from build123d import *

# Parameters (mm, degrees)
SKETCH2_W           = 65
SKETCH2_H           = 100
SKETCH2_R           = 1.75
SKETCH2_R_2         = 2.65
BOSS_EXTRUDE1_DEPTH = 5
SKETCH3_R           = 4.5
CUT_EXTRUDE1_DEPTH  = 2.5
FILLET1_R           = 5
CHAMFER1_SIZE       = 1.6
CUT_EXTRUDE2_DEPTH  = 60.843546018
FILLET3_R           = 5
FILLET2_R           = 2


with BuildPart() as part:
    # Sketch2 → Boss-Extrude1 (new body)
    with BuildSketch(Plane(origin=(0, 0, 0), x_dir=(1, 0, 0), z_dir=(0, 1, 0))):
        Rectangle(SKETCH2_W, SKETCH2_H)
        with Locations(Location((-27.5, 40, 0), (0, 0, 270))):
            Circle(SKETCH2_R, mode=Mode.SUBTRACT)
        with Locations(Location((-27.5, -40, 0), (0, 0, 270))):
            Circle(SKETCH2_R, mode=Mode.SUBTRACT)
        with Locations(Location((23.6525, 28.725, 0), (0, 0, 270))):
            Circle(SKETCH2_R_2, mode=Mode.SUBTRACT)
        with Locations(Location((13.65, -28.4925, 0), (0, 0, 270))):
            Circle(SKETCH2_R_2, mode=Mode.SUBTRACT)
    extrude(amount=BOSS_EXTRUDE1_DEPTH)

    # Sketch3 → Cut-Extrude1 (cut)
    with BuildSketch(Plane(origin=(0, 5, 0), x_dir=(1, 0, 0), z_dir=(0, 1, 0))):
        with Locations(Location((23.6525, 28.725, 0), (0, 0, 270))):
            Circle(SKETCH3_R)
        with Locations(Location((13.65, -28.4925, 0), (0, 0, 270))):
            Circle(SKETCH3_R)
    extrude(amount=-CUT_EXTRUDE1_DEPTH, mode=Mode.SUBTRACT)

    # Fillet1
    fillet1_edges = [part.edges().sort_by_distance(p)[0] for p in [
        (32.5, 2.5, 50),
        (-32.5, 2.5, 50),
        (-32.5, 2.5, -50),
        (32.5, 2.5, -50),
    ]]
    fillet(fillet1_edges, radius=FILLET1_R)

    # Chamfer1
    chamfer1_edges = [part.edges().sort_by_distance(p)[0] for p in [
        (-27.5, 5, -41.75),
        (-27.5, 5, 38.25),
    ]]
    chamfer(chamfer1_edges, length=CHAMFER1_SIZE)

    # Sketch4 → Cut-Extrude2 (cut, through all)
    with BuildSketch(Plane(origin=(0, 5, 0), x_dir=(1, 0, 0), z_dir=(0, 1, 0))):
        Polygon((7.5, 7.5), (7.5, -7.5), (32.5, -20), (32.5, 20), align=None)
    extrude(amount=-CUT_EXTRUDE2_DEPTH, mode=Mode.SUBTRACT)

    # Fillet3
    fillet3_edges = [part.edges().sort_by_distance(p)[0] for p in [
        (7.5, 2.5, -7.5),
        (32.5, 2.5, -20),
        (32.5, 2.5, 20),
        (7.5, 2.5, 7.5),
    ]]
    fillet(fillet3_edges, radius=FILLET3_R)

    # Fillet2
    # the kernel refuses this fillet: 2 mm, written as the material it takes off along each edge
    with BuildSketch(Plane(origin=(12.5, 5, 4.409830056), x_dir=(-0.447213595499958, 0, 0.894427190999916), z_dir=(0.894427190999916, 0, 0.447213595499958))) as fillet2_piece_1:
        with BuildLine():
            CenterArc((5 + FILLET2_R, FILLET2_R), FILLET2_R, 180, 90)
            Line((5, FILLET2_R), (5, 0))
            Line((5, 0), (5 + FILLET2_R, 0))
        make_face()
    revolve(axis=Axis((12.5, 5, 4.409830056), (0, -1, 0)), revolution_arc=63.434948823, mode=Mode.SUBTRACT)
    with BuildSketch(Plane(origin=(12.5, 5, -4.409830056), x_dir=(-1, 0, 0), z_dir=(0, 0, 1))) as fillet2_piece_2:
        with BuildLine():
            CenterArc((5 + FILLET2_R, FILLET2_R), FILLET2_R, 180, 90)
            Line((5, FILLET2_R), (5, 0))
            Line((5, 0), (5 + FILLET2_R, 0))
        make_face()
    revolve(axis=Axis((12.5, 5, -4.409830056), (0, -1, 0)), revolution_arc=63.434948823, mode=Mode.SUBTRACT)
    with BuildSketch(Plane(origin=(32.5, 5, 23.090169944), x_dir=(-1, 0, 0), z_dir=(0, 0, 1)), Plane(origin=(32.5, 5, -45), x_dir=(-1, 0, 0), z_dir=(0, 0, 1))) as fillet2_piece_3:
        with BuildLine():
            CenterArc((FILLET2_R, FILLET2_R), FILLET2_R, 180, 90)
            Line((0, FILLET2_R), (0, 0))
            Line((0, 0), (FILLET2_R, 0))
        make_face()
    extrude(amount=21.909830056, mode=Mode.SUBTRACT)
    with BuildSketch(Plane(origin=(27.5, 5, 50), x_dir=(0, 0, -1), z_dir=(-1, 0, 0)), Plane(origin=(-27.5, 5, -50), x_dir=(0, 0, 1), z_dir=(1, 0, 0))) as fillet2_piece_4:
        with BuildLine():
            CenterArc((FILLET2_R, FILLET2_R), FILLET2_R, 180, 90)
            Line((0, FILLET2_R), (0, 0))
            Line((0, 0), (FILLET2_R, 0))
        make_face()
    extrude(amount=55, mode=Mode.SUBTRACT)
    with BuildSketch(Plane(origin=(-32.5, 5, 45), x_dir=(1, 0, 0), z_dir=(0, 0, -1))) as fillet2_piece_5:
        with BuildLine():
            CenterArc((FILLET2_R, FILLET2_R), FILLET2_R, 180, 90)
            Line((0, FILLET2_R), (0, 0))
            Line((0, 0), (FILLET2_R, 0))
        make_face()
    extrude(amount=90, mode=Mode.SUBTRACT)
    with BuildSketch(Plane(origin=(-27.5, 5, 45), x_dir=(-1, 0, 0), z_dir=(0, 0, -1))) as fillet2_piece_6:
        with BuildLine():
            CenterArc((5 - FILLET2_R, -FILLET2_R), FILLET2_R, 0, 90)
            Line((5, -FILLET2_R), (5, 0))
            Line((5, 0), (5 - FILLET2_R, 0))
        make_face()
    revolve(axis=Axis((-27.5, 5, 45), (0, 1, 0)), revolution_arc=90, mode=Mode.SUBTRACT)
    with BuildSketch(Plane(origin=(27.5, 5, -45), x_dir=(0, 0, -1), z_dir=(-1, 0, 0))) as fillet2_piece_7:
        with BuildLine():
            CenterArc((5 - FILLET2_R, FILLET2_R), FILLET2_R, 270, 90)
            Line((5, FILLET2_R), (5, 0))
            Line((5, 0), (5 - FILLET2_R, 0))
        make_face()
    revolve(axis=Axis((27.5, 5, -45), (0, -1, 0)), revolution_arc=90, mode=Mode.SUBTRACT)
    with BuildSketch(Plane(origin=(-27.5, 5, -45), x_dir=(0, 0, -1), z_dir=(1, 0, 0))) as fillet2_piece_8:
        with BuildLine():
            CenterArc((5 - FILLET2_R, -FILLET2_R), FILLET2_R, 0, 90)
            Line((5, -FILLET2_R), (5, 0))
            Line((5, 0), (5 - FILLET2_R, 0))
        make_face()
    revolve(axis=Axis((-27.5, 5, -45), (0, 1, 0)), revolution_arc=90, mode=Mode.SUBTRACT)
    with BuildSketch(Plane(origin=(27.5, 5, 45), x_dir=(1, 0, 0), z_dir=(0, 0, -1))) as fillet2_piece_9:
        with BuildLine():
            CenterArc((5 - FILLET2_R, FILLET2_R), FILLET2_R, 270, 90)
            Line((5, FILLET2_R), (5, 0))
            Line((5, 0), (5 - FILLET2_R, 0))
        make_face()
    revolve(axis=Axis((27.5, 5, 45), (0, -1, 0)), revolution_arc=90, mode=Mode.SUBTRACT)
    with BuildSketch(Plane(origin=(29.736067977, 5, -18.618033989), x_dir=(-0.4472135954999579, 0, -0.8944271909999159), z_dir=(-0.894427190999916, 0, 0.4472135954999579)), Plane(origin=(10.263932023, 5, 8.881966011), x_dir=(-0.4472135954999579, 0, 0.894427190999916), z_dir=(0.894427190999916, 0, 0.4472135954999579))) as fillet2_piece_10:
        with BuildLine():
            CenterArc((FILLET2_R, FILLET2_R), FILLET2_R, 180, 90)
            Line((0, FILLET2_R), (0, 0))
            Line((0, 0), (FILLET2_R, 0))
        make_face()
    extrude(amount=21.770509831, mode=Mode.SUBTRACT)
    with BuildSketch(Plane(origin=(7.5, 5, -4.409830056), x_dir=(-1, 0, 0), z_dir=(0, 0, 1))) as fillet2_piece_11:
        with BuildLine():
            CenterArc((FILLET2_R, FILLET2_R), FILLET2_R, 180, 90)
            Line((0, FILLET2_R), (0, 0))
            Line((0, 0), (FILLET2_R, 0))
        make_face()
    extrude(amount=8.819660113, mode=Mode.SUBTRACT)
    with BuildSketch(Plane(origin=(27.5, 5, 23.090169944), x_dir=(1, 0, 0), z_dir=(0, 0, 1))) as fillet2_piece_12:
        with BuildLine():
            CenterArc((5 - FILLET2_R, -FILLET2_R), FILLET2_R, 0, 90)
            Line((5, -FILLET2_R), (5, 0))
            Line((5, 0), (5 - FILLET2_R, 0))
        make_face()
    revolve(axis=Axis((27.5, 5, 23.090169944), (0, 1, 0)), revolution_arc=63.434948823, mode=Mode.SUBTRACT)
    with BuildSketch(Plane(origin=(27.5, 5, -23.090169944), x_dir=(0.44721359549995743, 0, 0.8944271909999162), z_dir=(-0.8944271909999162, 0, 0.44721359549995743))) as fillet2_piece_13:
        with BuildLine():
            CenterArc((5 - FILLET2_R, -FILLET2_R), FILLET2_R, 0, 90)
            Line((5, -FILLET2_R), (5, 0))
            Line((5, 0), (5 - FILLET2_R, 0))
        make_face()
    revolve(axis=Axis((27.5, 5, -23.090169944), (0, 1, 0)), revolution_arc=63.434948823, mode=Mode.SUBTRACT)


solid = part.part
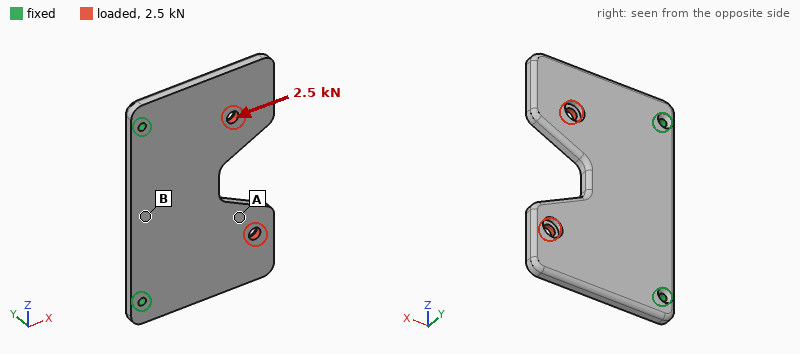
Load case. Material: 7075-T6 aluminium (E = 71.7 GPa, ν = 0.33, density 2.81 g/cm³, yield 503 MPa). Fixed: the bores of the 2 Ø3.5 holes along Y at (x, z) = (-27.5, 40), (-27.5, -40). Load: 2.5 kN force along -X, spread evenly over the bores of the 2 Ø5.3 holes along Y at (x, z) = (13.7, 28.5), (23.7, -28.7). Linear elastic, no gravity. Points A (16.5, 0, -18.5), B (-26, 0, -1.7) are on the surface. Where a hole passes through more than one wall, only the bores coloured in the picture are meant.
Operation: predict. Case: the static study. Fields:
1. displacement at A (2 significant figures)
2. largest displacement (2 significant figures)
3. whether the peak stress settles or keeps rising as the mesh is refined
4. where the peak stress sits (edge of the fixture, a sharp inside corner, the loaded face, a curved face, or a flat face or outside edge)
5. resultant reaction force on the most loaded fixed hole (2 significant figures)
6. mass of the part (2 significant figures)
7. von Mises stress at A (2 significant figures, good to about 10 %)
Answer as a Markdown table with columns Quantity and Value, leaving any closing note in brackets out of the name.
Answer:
| Quantity | Value |
|---|---|
| displacement at A | 0.073 mm |
| largest displacement | 0.12 mm |
| whether the peak stress settles or keeps rising as the mesh is refined | keeps rising |
| where the peak stress sits | edge of the fixture |
| resultant reaction force on the most loaded fixed hole | 1.3 kN |
| mass of the part | 79 g |
| von Mises stress at A | 17 MPa |
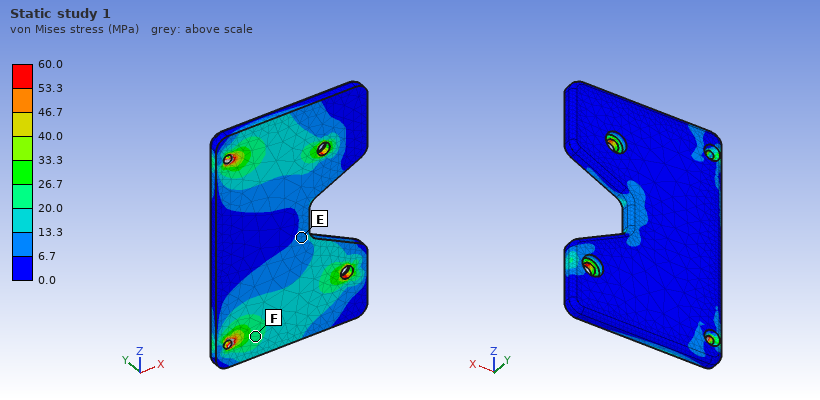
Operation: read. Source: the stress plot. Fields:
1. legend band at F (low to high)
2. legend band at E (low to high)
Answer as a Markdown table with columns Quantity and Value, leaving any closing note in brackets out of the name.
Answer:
| Quantity | Value |
|---|---|
| legend band at F | 20.0 to 26.7 MPa |
| legend band at E | 6.7 to 13.3 MPa |
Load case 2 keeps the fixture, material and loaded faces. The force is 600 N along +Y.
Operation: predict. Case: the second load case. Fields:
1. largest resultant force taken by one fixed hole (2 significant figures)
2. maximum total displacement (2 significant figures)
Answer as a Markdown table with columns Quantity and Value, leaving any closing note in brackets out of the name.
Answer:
| Quantity | Value |
|---|---|
| largest resultant force taken by one fixed hole | 300 N |
| maximum total displacement | 0.96 mm |
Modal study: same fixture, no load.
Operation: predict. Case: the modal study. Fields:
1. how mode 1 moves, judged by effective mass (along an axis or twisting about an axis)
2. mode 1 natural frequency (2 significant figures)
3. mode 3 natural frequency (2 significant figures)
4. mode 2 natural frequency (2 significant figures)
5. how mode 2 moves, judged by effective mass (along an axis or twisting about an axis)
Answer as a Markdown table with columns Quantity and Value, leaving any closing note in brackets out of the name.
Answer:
| Quantity | Value |
|---|---|
| how mode 1 moves, judged by effective mass | along Y |
| mode 1 natural frequency | 860 Hz |
| mode 3 natural frequency | 2800 Hz |
| mode 2 natural frequency | 1500 Hz |
| how mode 2 moves, judged by effective mass | twisting about X |
